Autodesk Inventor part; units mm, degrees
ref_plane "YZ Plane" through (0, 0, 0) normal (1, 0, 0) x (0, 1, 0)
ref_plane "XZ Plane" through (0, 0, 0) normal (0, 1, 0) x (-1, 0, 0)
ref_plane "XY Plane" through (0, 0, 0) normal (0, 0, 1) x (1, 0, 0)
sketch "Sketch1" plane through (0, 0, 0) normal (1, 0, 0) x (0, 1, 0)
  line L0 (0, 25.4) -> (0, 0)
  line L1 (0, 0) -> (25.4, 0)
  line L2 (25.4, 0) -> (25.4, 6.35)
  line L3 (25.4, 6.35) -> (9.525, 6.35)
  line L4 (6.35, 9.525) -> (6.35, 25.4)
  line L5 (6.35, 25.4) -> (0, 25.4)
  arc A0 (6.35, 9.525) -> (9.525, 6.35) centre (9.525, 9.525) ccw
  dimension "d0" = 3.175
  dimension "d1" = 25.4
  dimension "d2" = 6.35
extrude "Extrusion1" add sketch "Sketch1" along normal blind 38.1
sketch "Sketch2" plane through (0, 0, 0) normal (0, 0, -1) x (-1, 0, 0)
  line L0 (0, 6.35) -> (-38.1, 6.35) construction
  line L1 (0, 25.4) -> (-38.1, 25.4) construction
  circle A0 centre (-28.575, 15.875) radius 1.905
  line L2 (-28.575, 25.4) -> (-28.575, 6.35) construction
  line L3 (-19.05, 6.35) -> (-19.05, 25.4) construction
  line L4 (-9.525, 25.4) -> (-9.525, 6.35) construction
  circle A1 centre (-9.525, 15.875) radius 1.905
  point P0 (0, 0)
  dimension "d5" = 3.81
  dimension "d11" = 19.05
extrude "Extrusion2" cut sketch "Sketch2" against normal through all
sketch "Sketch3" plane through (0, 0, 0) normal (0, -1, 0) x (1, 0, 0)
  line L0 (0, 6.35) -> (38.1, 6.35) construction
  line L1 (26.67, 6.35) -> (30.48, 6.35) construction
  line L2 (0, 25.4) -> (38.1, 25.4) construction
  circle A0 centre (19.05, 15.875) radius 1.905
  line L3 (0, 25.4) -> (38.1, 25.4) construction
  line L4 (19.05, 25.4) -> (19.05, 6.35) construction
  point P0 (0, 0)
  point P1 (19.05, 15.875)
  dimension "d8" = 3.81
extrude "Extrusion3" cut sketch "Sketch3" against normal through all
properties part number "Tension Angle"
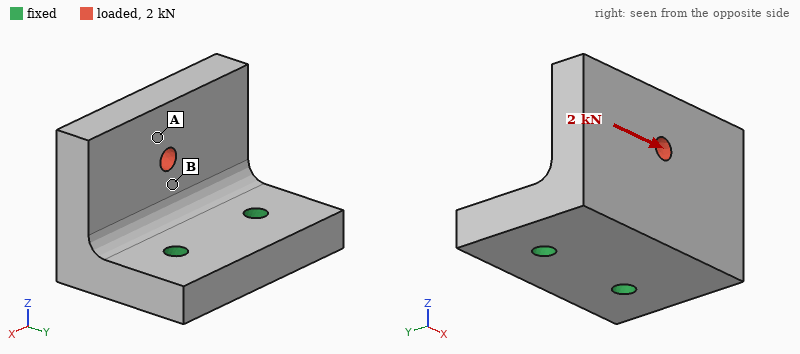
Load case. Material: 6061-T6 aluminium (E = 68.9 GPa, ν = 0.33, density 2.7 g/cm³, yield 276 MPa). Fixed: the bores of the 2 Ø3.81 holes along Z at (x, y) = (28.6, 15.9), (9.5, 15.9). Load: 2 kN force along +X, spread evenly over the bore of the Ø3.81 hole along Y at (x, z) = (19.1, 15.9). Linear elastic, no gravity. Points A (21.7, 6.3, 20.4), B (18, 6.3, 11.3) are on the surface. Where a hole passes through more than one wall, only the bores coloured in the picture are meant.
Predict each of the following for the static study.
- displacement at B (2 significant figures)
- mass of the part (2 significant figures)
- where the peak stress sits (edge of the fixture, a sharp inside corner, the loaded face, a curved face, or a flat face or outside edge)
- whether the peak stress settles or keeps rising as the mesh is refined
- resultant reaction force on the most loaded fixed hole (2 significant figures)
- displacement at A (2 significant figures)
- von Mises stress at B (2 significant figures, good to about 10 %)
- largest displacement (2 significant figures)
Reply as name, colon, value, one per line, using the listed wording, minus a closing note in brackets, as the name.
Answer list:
displacement at B: 18 µm
mass of the part: 29 g
where the peak stress sits: edge of the fixture
whether the peak stress settles or keeps rising as the mesh is refined: keeps rising
resultant reaction force on the most loaded fixed hole: 1.8 kN
displacement at A: 34 µm
von Mises stress at B: 41 MPa
largest displacement: 48 µm
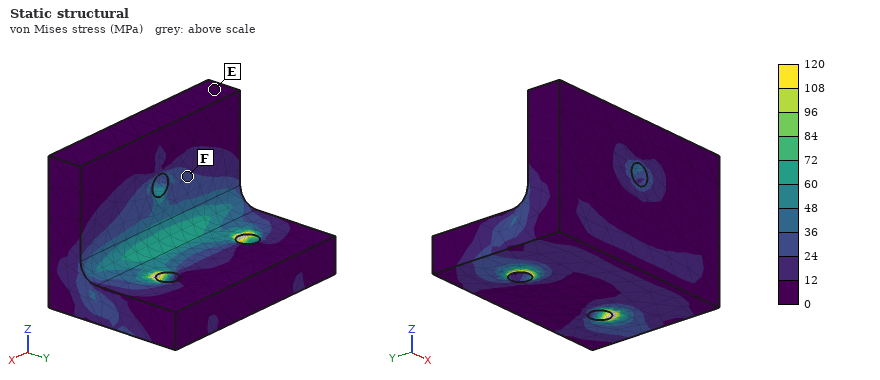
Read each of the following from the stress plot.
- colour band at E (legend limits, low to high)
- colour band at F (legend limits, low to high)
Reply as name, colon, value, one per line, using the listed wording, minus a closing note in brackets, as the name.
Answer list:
colour band at E: 0 to 12 MPa
colour band at F: 24 to 36 MPa
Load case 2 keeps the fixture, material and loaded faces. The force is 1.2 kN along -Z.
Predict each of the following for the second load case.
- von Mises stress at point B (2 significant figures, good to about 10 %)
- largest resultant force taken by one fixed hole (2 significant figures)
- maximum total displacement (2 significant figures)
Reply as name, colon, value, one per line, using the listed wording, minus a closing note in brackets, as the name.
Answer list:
von Mises stress at point B: 13 MPa
largest resultant force taken by one fixed hole: 600 N
maximum total displacement: 51 µm
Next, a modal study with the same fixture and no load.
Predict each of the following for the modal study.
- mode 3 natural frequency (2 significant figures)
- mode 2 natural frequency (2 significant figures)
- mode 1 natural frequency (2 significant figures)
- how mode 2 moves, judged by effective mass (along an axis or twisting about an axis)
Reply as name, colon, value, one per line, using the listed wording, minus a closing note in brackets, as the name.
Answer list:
mode 3 natural frequency: 15 kHz
mode 2 natural frequency: 9300 Hz
mode 1 natural frequency: 5600 Hz
how mode 2 moves, judged by effective mass: along X
